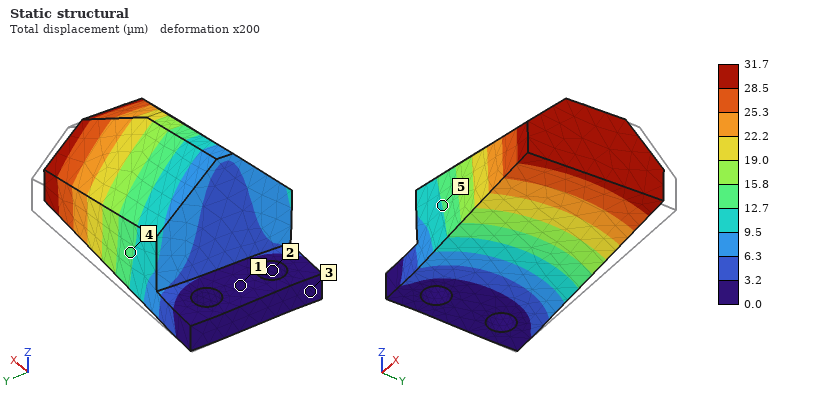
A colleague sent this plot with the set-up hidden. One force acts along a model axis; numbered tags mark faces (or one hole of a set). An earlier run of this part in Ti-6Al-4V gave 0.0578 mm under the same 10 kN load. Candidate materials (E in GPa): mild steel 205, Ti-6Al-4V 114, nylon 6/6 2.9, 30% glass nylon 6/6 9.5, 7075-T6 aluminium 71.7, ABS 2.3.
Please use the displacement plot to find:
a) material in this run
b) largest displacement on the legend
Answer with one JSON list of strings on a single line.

["mild steel", "31.7 µm"]
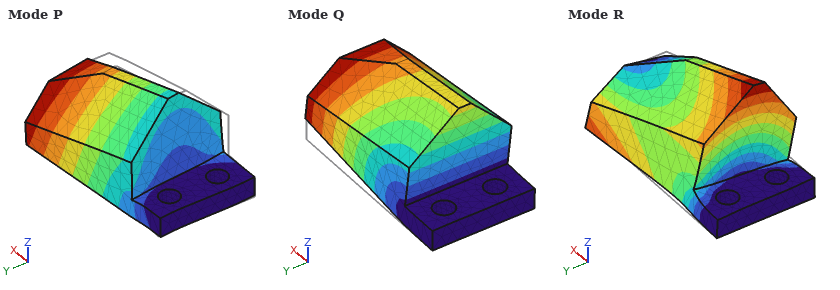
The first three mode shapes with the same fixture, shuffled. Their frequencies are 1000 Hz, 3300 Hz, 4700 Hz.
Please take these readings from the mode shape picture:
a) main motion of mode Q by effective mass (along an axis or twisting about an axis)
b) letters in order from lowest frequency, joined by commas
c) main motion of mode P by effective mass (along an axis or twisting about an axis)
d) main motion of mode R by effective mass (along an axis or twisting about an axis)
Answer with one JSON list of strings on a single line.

["along Z", "Q, P, R", "along Y", "twisting about X"]
